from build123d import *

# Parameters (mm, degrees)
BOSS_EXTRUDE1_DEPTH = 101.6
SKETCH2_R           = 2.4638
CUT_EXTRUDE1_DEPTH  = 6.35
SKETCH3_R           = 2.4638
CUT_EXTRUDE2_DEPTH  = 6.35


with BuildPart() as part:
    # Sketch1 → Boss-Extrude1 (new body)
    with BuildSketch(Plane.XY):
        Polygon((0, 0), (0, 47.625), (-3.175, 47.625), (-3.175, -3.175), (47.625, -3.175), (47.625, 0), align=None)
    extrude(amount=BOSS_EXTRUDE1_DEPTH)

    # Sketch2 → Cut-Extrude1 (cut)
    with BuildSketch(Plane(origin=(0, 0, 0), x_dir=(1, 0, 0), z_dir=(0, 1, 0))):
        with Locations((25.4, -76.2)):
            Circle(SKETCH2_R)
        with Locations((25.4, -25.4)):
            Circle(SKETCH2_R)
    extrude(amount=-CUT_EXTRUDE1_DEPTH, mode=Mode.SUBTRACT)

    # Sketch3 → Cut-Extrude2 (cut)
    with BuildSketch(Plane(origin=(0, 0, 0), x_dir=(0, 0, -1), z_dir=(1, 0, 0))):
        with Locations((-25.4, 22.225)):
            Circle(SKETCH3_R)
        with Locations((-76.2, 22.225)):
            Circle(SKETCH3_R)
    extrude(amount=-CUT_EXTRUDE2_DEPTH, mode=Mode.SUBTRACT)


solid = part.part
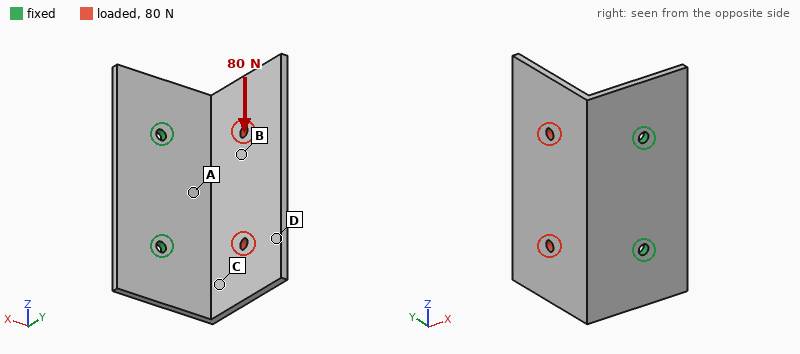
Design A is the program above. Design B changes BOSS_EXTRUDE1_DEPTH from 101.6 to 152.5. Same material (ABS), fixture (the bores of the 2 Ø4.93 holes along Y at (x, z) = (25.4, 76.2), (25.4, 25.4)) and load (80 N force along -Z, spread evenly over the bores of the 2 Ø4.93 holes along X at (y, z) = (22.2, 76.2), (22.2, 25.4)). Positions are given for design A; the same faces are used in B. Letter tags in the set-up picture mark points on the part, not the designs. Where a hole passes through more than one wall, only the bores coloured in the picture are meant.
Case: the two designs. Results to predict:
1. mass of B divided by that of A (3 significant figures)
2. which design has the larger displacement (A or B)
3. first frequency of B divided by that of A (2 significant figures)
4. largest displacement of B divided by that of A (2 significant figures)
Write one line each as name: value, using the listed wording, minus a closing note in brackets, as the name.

mass of B divided by that of A: 1.50
which design has the larger displacement: B
first frequency of B divided by that of A: 0.81
largest displacement of B divided by that of A: 1.4
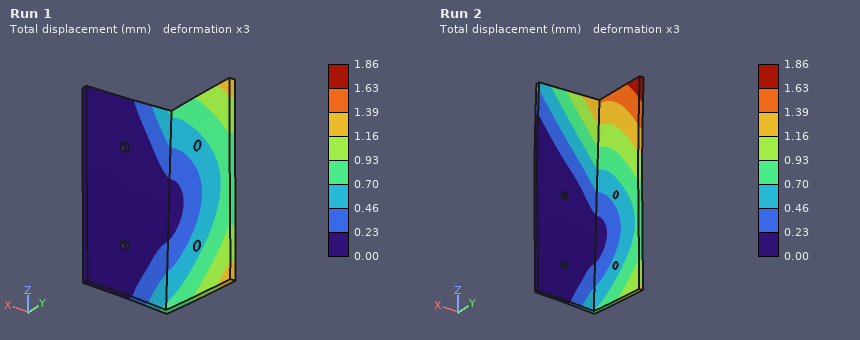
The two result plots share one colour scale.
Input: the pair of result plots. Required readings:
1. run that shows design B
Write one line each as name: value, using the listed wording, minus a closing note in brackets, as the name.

run that shows design B: Run 2
